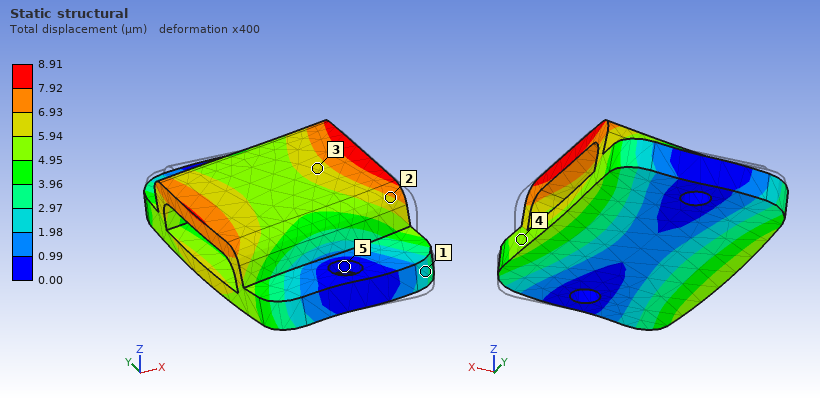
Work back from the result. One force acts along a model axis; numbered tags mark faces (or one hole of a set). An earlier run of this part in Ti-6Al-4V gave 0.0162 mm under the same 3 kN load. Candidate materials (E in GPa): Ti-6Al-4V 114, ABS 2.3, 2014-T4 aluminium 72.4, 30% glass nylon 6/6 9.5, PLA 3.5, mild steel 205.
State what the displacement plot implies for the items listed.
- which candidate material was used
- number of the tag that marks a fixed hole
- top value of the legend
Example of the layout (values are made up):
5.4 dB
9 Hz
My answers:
mild steel
5
8.91 µm
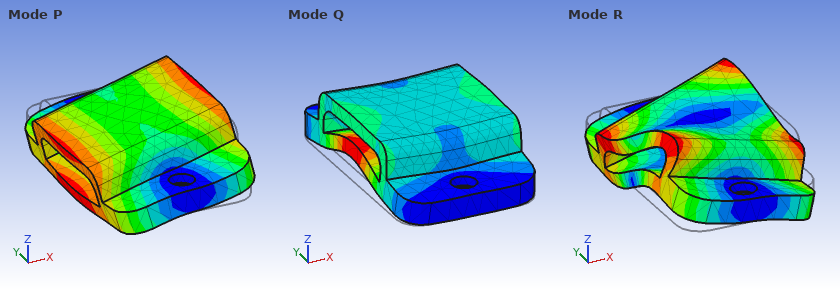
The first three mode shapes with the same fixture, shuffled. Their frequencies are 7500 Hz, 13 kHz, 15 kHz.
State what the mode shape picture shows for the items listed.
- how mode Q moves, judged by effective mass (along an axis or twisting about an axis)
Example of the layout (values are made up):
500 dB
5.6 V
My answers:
along Z
